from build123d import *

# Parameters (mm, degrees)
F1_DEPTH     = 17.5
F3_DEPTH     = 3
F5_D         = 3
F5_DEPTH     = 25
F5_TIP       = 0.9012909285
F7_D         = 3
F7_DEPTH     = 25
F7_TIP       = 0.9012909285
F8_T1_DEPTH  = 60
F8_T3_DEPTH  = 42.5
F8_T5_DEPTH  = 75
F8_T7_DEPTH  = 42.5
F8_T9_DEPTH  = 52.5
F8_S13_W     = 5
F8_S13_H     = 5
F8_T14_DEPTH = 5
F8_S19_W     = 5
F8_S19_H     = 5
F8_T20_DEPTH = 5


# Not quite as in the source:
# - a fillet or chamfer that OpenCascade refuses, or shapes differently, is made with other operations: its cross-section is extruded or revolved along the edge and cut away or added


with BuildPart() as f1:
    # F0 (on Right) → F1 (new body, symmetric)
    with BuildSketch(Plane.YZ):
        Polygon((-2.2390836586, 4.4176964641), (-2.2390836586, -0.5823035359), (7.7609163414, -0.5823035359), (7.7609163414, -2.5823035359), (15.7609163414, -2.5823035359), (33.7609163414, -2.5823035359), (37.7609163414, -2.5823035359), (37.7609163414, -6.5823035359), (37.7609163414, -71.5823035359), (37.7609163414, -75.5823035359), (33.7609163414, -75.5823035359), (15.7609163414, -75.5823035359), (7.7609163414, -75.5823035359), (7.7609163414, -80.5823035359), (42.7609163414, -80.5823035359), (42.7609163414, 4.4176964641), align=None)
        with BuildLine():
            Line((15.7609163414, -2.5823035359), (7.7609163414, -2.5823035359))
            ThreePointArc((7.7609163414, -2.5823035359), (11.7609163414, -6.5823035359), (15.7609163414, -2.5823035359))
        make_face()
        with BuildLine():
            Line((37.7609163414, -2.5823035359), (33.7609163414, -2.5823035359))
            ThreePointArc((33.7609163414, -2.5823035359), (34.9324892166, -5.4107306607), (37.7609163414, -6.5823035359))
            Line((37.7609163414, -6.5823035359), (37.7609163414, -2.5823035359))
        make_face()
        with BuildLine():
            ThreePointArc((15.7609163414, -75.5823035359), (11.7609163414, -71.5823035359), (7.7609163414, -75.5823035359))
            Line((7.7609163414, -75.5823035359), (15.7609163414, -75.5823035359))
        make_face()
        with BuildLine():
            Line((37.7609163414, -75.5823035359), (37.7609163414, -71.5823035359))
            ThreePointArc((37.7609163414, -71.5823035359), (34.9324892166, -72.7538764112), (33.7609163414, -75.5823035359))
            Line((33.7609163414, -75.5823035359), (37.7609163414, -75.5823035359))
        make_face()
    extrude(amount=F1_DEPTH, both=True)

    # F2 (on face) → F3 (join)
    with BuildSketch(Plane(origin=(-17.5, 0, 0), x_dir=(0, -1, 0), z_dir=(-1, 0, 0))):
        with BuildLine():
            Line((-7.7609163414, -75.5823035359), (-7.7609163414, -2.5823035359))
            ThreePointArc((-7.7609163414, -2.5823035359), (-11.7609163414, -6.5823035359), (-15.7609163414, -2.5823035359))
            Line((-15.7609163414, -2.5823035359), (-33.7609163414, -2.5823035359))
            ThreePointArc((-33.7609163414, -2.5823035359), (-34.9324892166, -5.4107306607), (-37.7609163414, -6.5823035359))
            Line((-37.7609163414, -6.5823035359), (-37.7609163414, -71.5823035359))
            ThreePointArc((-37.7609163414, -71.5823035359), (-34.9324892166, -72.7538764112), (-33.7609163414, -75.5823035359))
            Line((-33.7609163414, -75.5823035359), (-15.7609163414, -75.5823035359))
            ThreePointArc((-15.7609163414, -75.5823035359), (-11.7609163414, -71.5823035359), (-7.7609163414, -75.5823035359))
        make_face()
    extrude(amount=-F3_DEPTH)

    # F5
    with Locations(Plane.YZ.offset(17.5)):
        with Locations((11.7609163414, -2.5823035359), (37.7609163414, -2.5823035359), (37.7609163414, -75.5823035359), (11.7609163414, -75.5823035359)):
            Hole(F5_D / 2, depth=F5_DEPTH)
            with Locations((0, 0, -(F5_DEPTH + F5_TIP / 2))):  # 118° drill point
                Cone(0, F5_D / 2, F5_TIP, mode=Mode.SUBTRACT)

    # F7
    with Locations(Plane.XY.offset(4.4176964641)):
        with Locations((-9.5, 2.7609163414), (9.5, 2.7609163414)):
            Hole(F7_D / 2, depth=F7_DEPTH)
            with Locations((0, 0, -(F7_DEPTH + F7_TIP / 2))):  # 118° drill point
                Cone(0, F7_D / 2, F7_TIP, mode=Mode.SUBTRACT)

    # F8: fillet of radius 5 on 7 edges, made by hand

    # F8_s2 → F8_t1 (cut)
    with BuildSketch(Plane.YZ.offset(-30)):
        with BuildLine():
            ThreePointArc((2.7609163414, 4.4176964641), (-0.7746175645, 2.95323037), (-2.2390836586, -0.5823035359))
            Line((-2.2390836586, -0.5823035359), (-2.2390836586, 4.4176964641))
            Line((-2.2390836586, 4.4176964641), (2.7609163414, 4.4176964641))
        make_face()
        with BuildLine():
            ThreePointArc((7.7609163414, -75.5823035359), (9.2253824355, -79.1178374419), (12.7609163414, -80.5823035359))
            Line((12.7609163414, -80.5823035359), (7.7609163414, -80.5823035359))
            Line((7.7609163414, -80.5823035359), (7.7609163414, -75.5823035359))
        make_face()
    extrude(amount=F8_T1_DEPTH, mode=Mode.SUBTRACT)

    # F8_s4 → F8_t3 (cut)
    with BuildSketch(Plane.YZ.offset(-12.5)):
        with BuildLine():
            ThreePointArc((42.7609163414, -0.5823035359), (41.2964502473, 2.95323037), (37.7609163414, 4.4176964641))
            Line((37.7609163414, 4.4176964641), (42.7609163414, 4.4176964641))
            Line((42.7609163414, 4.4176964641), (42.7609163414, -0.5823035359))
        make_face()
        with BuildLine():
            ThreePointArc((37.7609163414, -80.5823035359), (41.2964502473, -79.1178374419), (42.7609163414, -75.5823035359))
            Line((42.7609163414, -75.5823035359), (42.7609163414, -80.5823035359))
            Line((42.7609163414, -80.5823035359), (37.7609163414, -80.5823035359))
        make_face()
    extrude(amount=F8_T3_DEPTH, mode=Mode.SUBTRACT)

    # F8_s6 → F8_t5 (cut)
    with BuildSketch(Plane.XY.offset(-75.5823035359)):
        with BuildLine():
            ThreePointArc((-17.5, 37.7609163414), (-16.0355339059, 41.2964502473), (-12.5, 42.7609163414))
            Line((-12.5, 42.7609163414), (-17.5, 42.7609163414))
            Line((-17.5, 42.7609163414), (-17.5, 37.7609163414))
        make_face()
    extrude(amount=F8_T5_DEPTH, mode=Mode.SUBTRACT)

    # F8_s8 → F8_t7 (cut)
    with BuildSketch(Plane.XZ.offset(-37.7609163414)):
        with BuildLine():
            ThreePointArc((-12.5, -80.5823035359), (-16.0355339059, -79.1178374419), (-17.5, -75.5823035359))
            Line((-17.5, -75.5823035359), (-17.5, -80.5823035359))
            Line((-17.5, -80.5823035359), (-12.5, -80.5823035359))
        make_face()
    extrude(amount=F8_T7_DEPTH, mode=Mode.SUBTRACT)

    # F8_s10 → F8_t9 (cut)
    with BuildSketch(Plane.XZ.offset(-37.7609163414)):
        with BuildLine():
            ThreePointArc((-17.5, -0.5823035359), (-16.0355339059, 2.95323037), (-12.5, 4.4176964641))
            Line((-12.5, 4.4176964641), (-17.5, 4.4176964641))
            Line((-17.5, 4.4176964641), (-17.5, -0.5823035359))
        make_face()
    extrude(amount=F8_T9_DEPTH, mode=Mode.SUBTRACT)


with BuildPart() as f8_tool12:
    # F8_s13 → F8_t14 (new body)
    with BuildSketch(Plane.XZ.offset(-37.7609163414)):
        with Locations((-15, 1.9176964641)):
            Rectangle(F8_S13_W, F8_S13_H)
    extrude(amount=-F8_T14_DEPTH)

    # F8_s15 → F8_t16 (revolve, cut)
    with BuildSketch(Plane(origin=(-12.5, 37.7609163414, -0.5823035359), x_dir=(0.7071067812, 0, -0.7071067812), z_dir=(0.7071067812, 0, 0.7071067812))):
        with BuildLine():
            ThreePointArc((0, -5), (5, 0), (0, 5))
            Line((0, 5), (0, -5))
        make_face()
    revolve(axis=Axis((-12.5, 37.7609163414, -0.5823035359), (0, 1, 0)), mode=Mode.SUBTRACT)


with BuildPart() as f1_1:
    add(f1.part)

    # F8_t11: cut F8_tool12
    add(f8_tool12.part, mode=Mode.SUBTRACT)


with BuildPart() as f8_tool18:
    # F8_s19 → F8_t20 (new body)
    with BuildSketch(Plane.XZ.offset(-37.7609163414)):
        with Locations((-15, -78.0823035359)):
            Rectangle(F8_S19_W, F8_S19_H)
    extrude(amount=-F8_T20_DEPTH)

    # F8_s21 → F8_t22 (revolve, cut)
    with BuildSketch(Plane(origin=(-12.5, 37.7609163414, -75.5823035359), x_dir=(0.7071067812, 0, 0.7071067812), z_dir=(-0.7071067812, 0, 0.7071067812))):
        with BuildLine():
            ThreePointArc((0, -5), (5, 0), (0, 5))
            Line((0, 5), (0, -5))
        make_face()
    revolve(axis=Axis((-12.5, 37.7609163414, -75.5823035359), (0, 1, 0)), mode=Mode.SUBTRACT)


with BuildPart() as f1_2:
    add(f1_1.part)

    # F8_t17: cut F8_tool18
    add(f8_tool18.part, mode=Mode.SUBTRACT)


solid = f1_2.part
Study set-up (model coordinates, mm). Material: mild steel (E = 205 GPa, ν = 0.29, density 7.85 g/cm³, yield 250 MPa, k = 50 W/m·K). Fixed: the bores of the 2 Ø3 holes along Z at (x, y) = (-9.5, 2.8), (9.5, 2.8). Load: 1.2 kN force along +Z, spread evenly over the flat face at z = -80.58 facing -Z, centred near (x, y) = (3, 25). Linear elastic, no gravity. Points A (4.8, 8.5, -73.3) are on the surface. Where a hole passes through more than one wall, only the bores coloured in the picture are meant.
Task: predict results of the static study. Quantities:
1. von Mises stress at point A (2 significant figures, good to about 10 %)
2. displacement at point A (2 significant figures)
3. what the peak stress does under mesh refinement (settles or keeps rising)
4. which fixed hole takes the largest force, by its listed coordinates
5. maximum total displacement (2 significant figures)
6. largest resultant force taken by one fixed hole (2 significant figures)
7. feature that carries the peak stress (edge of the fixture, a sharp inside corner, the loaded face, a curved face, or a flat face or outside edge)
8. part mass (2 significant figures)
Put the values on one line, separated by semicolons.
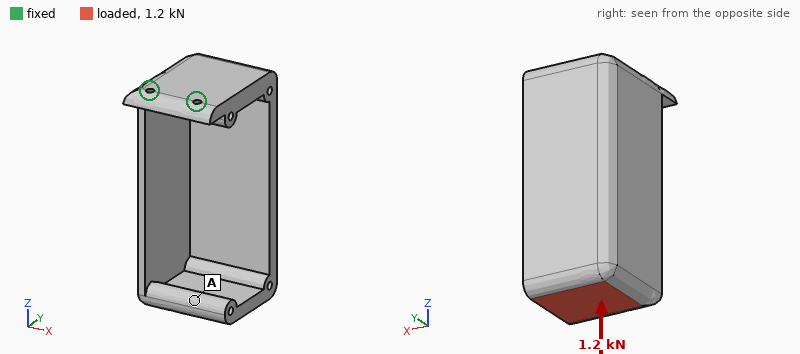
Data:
16 MPa; 0.22 mm; keeps rising; (9.5, 2.8); 0.26 mm; 730 N; edge of the fixture; 280 g
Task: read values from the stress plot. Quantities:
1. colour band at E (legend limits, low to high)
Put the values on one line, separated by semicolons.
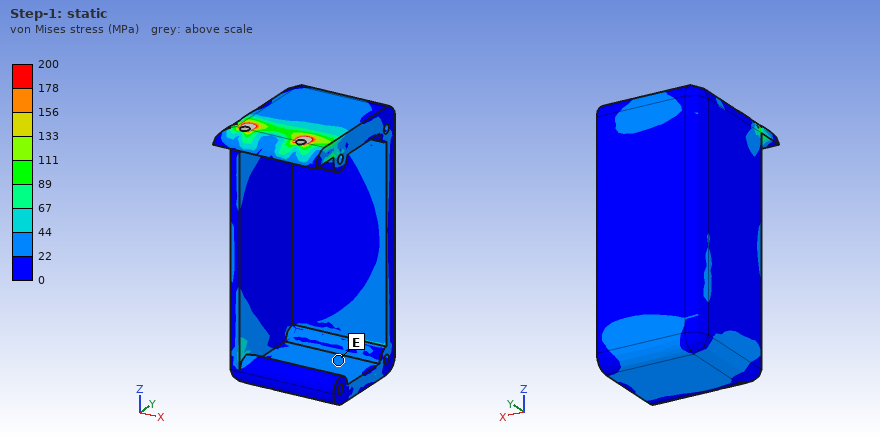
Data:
22 to 44 MPa
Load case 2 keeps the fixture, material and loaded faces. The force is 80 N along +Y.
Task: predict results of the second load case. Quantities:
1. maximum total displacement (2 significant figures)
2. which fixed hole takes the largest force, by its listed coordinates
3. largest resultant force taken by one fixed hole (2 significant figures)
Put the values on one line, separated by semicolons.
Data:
0.12 mm; (9.5, 2.8); 79 N
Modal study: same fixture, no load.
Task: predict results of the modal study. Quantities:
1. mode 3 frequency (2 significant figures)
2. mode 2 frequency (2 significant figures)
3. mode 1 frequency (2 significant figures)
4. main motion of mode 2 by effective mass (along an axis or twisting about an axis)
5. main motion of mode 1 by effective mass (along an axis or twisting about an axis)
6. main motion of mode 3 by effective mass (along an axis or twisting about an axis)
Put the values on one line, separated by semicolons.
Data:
1600 Hz; 630 Hz; 420 Hz; along X; along Y; along Z
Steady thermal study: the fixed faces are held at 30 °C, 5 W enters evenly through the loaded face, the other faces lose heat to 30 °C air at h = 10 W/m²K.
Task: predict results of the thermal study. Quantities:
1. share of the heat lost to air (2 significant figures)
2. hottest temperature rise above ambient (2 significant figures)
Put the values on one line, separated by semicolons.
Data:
48 %; 30 K
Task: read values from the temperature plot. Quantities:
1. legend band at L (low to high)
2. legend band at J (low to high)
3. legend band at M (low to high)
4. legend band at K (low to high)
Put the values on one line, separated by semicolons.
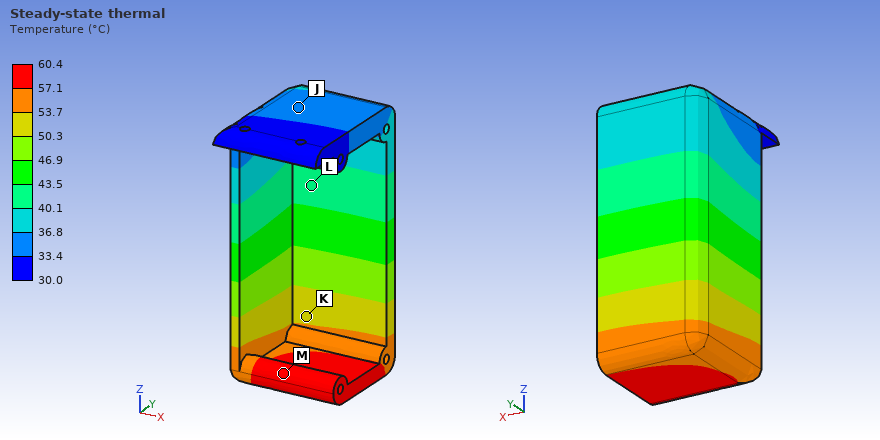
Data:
40.1 to 43.5 °C; 33.4 to 36.8 °C; 57.1 to 60.4 °C; 50.3 to 53.7 °C
